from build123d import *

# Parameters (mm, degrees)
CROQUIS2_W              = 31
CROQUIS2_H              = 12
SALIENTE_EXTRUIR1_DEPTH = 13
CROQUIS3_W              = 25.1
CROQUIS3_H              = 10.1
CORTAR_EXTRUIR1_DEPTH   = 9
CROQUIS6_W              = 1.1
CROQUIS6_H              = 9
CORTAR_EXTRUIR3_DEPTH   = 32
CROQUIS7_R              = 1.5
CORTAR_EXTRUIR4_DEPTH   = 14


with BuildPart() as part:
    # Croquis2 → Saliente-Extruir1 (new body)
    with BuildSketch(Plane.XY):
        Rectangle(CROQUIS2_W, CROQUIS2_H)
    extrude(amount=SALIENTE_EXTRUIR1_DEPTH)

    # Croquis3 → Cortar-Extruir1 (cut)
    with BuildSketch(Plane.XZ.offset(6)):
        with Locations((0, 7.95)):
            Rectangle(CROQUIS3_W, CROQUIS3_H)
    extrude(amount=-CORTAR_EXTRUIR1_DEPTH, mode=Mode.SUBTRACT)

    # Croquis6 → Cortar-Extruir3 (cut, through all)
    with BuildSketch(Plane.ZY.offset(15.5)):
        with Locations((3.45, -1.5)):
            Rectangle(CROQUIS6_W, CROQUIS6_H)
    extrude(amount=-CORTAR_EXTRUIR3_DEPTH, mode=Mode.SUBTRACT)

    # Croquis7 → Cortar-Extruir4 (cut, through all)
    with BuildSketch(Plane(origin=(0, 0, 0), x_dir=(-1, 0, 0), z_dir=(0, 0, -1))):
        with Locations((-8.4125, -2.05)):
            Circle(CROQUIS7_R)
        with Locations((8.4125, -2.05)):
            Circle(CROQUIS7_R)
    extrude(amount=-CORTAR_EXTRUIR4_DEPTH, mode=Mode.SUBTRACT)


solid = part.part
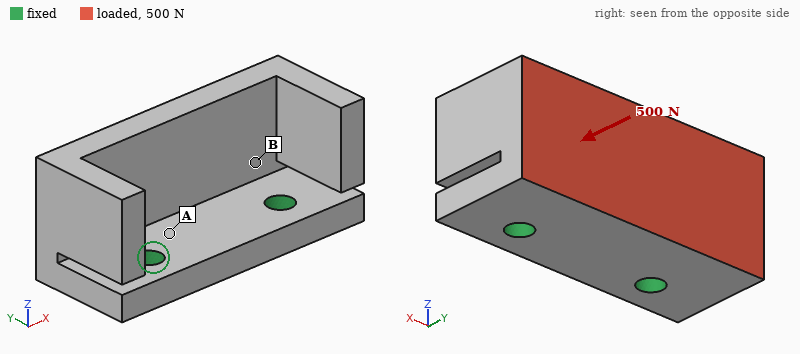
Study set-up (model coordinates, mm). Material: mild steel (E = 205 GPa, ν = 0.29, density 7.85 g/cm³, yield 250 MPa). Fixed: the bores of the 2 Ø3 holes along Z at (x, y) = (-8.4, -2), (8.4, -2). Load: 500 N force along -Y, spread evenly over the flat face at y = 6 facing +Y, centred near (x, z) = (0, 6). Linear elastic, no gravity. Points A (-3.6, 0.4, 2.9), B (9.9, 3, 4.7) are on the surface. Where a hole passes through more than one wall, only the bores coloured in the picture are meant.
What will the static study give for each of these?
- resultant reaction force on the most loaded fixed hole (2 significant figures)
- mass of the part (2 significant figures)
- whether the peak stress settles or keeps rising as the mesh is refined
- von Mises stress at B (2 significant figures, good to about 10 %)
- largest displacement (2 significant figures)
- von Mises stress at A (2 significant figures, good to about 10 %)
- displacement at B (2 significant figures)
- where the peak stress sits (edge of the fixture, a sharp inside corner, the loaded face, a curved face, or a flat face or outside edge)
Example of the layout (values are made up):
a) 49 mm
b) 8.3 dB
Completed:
a) 250 N
b) 19 g
c) keeps rising
d) 21 MPa
e) 23 µm
f) 44 MPa
g) 5.1 µm
h) edge of the fixture
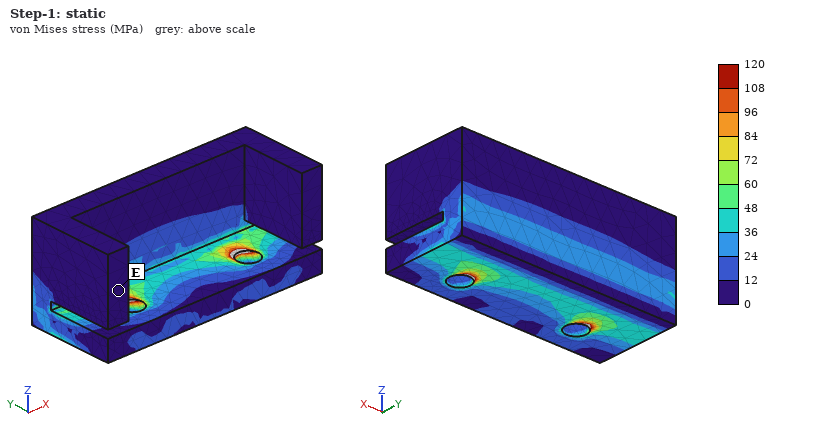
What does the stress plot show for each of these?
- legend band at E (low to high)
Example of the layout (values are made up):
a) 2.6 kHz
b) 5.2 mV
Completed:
a) 0 to 12 MPa
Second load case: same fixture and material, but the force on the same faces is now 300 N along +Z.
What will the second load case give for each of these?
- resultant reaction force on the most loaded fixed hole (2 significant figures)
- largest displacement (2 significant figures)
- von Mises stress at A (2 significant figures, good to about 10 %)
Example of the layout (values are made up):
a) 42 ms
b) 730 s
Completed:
a) 150 N
b) 11 µm
c) 24 MPa
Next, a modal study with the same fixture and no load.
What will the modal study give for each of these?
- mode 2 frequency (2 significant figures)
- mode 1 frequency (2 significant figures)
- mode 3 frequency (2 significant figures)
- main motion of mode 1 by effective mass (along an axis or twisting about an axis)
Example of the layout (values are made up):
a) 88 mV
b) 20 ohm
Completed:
a) 9400 Hz
b) 7200 Hz
c) 14 kHz
d) along Y
